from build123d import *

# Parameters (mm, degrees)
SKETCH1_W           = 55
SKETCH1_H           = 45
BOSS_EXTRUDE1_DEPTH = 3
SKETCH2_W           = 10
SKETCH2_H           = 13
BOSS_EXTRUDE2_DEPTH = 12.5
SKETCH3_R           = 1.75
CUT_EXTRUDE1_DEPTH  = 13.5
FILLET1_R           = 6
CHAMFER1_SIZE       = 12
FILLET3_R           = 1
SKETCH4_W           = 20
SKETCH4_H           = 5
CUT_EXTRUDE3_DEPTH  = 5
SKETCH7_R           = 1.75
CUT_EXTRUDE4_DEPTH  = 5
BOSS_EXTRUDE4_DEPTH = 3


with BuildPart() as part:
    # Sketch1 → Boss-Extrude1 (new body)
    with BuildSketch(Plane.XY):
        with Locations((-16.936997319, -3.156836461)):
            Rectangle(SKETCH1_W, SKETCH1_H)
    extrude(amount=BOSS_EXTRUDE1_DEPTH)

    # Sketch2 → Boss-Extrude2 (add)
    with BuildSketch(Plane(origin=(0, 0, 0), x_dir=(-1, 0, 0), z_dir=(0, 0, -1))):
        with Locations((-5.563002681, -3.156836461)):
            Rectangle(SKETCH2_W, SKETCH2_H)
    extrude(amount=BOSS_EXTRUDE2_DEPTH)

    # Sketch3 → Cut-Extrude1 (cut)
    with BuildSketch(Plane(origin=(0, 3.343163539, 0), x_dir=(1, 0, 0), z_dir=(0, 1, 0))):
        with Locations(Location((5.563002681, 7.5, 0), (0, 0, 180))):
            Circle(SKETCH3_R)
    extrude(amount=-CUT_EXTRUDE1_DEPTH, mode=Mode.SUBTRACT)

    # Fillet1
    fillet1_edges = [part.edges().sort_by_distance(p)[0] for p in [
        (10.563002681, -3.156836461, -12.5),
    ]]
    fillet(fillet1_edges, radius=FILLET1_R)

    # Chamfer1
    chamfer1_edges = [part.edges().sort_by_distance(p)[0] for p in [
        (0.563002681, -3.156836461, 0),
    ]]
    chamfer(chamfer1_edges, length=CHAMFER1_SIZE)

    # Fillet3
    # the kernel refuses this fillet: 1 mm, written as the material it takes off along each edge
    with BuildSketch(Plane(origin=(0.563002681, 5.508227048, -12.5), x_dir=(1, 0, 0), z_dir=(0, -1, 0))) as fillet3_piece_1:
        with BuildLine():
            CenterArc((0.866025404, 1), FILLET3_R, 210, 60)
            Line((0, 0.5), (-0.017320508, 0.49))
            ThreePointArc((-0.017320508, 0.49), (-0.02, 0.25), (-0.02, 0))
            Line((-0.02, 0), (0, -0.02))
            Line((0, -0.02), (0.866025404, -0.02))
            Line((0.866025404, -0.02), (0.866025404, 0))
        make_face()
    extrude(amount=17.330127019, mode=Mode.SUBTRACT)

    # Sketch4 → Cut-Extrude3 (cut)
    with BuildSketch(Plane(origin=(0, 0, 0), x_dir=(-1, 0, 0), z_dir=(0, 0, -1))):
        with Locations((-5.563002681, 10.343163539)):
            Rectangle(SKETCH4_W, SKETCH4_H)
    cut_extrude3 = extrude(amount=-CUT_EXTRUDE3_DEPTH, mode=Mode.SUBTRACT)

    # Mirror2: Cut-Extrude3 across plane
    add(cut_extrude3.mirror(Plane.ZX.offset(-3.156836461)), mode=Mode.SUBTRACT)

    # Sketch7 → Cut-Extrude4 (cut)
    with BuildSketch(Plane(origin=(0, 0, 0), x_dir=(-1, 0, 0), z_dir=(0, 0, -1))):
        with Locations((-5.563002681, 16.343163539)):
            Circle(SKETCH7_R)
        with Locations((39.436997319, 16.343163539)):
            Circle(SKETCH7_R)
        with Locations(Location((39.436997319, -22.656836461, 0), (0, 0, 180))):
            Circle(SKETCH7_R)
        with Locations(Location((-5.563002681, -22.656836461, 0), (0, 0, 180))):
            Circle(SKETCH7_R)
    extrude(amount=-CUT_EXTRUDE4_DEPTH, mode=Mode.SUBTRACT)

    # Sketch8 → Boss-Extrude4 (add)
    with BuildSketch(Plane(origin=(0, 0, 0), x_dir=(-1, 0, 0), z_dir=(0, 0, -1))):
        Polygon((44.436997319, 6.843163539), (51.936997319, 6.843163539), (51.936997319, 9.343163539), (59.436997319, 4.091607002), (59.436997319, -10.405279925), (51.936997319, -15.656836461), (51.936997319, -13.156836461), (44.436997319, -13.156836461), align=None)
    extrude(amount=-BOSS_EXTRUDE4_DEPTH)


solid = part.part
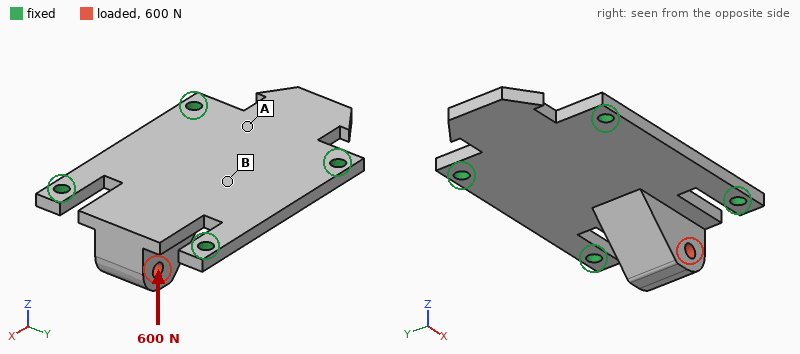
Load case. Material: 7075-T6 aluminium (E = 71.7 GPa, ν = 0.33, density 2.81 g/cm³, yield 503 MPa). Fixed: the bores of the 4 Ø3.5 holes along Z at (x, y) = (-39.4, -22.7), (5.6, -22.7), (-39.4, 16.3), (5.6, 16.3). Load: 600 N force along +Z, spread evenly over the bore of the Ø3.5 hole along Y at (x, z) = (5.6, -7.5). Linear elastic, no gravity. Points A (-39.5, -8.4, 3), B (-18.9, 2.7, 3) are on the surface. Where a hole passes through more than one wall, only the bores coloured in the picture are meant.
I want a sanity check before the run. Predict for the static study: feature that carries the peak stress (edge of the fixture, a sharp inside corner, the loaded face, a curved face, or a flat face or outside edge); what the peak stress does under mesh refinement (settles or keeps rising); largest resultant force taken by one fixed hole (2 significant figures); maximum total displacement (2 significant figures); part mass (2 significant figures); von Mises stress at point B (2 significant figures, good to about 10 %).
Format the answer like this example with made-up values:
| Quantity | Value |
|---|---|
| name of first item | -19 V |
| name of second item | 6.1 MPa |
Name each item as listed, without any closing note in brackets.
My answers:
| Quantity | Value |
|---|---|
| feature that carries the peak stress | edge of the fixture |
| what the peak stress does under mesh refinement | keeps rising |
| largest resultant force taken by one fixed hole | 350 N |
| maximum total displacement | 0.42 mm |
| part mass | 28 g |
| von Mises stress at point B | 48 MPa |
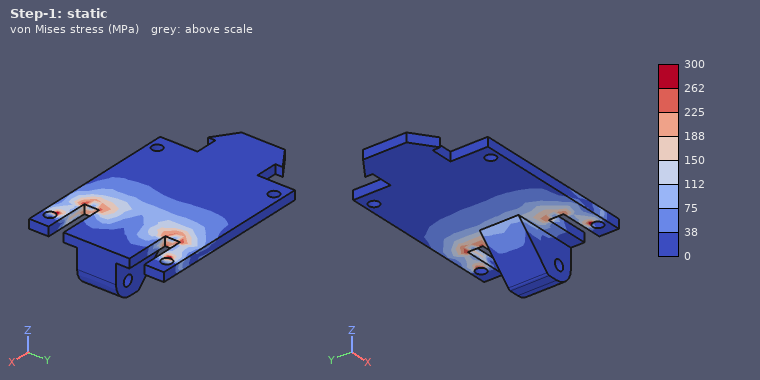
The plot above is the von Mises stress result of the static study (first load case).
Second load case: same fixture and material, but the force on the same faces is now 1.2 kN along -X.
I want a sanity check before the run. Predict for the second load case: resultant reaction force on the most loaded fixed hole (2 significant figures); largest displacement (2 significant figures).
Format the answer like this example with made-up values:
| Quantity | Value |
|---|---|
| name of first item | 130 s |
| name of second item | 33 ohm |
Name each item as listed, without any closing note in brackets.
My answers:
| Quantity | Value |
|---|---|
| resultant reaction force on the most loaded fixed hole | 480 N |
| largest displacement | 0.36 mm |
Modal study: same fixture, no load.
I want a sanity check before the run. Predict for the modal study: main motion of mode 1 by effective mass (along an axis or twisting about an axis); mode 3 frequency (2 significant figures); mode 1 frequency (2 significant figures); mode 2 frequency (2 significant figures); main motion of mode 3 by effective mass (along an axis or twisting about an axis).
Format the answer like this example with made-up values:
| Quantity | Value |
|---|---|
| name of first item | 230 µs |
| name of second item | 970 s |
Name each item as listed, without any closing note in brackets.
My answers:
| Quantity | Value |
|---|---|
| main motion of mode 1 by effective mass | along Z |
| mode 3 frequency | 5300 Hz |
| mode 1 frequency | 2400 Hz |
| mode 2 frequency | 4200 Hz |
| main motion of mode 3 by effective mass | along Z |
